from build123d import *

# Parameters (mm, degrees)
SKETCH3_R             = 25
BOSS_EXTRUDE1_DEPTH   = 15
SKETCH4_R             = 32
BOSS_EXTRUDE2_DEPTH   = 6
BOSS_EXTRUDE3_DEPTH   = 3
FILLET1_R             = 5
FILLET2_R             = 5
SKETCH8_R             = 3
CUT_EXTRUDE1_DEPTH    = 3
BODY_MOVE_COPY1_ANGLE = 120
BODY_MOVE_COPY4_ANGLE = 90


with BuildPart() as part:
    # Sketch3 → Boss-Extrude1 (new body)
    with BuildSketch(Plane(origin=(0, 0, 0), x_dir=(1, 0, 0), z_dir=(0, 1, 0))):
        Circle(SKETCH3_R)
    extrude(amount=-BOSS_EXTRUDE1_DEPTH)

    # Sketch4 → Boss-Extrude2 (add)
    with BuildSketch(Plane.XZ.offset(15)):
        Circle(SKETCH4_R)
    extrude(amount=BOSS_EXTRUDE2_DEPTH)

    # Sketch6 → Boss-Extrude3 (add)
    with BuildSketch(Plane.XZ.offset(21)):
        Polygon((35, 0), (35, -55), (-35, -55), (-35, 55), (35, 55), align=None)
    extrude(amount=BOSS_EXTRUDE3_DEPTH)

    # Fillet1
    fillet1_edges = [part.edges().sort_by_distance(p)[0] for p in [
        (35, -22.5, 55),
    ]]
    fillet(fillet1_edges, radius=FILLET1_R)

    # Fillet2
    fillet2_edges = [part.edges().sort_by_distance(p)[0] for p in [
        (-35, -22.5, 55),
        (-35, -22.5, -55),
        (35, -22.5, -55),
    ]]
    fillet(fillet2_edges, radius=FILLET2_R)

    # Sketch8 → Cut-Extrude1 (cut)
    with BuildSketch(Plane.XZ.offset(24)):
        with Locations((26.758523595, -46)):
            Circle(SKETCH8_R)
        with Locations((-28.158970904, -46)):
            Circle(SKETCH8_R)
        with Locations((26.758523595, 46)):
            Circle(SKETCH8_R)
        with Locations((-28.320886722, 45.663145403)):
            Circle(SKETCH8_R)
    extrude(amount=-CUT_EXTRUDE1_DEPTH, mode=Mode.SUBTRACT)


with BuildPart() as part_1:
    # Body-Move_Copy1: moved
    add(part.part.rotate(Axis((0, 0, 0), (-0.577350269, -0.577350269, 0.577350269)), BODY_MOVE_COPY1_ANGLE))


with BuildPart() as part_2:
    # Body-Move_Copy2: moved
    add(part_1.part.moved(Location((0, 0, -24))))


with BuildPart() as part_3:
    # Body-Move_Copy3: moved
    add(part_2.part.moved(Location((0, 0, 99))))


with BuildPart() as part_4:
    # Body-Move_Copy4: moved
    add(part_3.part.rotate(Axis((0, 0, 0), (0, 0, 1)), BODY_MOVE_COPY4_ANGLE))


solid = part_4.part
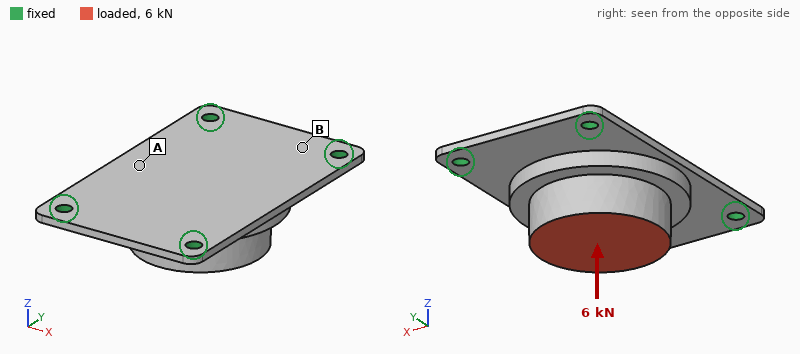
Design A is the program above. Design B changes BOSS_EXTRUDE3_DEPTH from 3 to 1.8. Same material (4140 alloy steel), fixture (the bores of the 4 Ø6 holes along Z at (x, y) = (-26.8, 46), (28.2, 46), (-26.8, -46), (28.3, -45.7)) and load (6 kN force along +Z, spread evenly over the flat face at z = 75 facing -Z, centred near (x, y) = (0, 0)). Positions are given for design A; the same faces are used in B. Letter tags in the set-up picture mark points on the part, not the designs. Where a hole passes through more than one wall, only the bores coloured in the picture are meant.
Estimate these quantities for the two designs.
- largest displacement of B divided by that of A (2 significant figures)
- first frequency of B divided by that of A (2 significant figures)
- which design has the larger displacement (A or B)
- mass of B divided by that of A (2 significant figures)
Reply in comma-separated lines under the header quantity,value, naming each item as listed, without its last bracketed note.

quantity,value
largest displacement of B divided by that of A,3.8
first frequency of B divided by that of A,0.54
which design has the larger displacement,B
mass of B divided by that of A,0.87
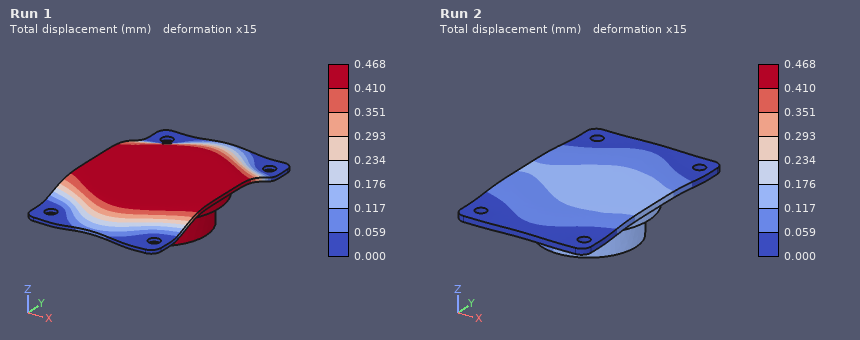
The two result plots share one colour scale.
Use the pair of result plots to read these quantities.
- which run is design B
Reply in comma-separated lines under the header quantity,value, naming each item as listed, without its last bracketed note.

quantity,value
which run is design B,Run 1
